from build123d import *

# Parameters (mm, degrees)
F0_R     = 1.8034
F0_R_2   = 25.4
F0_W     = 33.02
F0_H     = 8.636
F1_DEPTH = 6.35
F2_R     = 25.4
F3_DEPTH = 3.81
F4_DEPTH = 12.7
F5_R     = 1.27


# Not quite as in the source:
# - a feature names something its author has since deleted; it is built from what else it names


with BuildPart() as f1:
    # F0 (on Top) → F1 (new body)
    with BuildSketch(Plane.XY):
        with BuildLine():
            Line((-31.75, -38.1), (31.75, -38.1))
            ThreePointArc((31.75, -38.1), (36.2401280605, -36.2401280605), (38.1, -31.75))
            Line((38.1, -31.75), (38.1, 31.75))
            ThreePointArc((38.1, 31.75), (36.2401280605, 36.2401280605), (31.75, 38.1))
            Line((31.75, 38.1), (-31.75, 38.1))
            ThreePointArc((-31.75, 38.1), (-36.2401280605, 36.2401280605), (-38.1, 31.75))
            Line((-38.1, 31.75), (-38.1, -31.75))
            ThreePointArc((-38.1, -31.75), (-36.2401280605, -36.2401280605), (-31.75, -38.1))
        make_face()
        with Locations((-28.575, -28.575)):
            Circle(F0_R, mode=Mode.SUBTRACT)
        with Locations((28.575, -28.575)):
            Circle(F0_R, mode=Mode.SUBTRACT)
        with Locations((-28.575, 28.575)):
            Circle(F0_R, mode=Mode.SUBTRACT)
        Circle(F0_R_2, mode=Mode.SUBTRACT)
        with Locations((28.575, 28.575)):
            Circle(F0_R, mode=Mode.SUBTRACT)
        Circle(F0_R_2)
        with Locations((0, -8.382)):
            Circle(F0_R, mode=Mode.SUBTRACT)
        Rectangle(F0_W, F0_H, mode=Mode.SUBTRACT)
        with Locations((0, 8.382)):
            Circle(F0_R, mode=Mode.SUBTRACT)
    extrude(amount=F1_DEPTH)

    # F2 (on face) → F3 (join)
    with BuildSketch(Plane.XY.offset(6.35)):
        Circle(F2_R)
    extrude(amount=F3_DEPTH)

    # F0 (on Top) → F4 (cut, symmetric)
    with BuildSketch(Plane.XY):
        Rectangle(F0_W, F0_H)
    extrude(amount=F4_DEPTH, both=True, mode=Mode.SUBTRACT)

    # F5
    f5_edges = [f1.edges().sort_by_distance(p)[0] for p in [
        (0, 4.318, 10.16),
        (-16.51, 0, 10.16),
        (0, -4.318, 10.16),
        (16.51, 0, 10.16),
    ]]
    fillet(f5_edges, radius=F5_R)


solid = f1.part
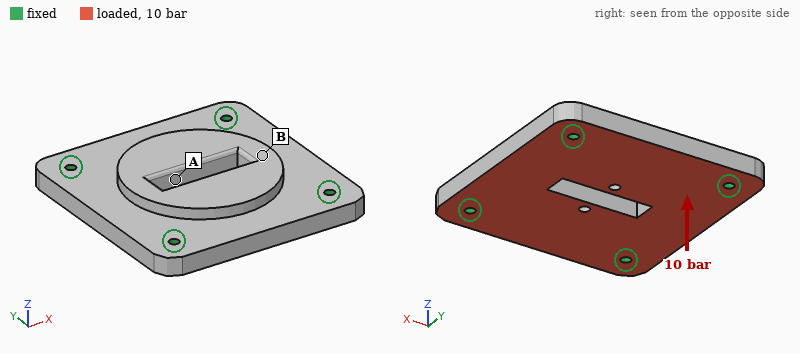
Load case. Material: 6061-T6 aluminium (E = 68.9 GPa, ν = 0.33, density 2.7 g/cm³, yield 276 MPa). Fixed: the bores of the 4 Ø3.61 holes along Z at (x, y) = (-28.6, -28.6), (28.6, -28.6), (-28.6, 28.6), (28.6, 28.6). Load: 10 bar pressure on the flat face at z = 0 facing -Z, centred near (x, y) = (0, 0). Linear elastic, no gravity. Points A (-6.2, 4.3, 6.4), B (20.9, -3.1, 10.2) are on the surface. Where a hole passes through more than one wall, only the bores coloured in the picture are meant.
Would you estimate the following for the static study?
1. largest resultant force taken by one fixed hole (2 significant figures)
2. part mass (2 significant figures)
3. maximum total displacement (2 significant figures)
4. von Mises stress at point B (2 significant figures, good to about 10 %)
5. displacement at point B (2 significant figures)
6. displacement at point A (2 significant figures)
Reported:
1.4 kN
110 g
39 µm
25 MPa
30 µm
38 µm
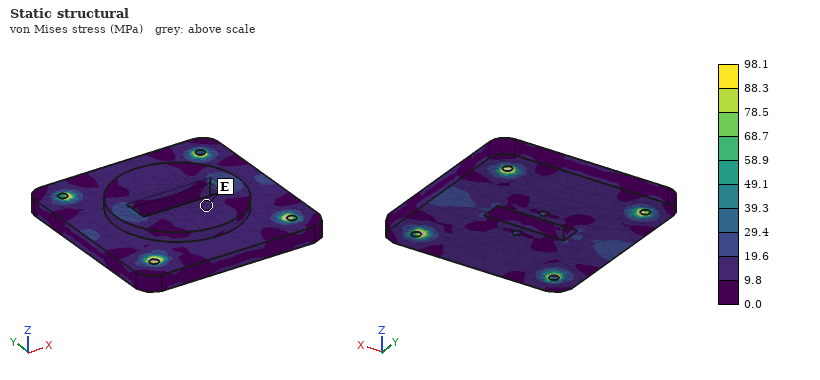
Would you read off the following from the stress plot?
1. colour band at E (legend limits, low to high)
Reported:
9.8 to 19.6 MPa
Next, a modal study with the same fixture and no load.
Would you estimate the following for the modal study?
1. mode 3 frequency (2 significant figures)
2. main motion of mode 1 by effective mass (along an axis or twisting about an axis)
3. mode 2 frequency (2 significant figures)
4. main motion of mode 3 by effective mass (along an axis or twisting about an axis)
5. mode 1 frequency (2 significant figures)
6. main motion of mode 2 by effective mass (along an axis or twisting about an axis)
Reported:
10 kHz
along Z
9600 Hz
twisting about Y
6400 Hz
twisting about X
